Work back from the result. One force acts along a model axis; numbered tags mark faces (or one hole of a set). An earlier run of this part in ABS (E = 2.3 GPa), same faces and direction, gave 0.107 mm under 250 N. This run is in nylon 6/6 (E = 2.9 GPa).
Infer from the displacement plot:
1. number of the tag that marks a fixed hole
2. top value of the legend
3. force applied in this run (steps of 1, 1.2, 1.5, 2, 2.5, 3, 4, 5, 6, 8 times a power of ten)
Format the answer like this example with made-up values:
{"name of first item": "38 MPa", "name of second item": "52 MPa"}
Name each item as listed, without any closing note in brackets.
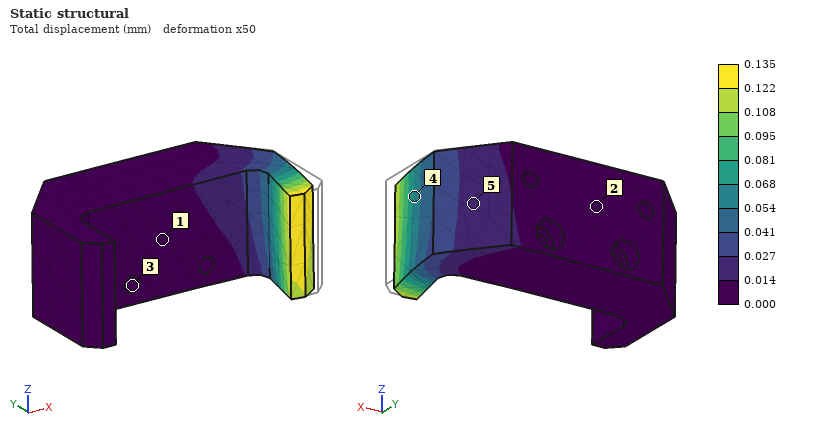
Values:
{"number of the tag that marks a fixed hole": "3", "top value of the legend": "0.135 mm", "force applied in this run": "400 N"}
